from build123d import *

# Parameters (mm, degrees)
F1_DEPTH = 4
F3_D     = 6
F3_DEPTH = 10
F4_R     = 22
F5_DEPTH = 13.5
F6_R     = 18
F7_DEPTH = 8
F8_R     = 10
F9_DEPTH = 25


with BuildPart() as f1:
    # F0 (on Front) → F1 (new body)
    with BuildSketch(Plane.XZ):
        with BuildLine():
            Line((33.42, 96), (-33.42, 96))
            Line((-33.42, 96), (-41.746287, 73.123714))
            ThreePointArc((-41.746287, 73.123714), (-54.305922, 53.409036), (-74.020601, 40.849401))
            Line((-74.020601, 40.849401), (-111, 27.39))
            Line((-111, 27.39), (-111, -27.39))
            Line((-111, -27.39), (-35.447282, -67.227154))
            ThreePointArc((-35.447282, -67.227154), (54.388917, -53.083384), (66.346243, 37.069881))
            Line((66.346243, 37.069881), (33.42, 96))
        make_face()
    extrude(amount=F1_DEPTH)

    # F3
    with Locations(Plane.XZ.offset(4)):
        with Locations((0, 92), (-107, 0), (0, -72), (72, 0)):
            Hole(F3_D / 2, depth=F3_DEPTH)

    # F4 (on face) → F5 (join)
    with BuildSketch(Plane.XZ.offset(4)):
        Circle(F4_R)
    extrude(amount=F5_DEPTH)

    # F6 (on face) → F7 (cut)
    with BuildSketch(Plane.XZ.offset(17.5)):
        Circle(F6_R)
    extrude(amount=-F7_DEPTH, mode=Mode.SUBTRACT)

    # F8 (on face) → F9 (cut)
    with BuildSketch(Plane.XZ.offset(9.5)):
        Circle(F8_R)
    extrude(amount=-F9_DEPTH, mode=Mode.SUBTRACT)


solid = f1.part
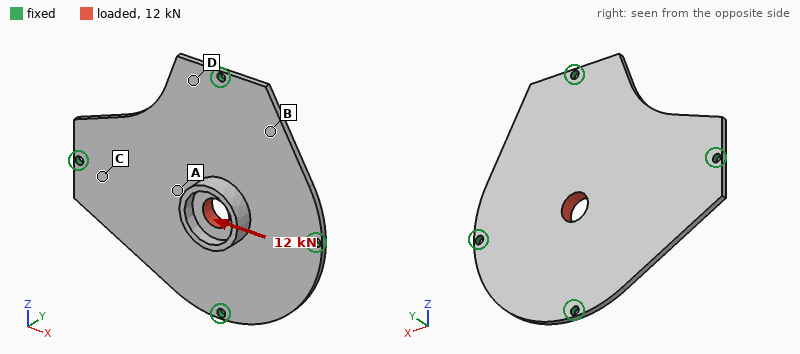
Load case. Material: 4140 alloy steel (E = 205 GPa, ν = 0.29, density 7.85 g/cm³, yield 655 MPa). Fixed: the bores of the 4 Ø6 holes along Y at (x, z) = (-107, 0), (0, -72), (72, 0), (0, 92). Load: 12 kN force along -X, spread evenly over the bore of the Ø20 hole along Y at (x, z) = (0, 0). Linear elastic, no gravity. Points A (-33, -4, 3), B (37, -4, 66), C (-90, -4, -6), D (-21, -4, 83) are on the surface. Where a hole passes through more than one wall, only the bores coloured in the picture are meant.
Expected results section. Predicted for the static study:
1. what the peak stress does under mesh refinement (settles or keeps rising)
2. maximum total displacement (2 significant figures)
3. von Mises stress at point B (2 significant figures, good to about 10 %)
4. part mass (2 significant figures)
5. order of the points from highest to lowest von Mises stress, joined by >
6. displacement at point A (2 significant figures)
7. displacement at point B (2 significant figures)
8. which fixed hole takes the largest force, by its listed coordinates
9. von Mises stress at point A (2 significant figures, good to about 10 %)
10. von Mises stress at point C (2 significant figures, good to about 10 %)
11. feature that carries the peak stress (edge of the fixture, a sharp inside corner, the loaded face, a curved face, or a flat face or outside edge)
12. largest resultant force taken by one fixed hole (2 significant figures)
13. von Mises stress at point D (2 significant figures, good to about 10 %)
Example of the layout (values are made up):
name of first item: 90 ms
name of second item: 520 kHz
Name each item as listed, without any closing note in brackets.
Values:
what the peak stress does under mesh refinement: keeps rising
maximum total displacement: 67 µm
von Mises stress at point B: 8.0 MPa
part mass: 800 g
order of the points from highest to lowest von Mises stress, joined by >: A > C > D > B
displacement at point A: 65 µm
displacement at point B: 14 µm
which fixed hole takes the largest force, by its listed coordinates: (72, 0)
von Mises stress at point A: 57 MPa
von Mises stress at point C: 25 MPa
feature that carries the peak stress: edge of the fixture
largest resultant force taken by one fixed hole: 4.4 kN
von Mises stress at point D: 15 MPa
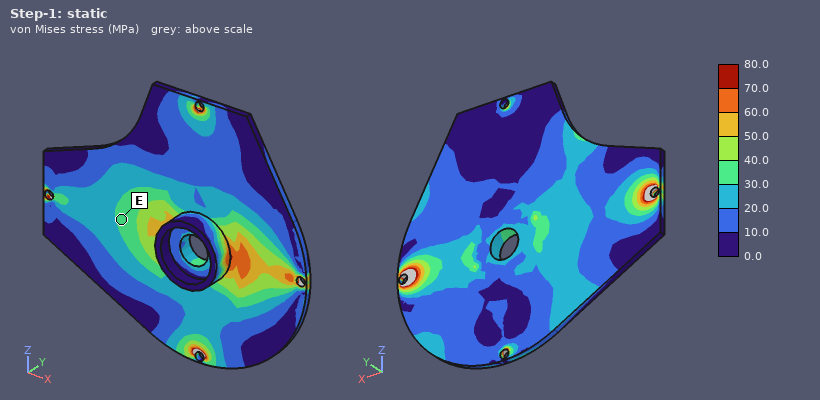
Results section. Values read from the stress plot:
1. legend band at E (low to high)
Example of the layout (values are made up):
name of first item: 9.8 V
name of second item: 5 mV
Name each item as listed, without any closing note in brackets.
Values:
legend band at E: 30.0 to 40.0 MPa
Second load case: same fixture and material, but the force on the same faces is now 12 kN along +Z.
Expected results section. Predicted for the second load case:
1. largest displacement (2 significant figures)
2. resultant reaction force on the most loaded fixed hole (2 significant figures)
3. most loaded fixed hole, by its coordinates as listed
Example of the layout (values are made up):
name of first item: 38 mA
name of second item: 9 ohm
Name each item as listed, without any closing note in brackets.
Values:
largest displacement: 58 µm
resultant reaction force on the most loaded fixed hole: 4.6 kN
most loaded fixed hole, by its coordinates as listed: (0, -72)
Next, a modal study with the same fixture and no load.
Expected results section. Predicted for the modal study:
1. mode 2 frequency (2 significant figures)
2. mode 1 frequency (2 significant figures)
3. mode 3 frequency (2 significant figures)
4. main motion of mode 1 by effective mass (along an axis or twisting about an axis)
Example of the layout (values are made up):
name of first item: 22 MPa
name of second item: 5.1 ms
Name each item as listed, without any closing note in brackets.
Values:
mode 2 frequency: 1400 Hz
mode 1 frequency: 840 Hz
mode 3 frequency: 1400 Hz
main motion of mode 1 by effective mass: along Y
